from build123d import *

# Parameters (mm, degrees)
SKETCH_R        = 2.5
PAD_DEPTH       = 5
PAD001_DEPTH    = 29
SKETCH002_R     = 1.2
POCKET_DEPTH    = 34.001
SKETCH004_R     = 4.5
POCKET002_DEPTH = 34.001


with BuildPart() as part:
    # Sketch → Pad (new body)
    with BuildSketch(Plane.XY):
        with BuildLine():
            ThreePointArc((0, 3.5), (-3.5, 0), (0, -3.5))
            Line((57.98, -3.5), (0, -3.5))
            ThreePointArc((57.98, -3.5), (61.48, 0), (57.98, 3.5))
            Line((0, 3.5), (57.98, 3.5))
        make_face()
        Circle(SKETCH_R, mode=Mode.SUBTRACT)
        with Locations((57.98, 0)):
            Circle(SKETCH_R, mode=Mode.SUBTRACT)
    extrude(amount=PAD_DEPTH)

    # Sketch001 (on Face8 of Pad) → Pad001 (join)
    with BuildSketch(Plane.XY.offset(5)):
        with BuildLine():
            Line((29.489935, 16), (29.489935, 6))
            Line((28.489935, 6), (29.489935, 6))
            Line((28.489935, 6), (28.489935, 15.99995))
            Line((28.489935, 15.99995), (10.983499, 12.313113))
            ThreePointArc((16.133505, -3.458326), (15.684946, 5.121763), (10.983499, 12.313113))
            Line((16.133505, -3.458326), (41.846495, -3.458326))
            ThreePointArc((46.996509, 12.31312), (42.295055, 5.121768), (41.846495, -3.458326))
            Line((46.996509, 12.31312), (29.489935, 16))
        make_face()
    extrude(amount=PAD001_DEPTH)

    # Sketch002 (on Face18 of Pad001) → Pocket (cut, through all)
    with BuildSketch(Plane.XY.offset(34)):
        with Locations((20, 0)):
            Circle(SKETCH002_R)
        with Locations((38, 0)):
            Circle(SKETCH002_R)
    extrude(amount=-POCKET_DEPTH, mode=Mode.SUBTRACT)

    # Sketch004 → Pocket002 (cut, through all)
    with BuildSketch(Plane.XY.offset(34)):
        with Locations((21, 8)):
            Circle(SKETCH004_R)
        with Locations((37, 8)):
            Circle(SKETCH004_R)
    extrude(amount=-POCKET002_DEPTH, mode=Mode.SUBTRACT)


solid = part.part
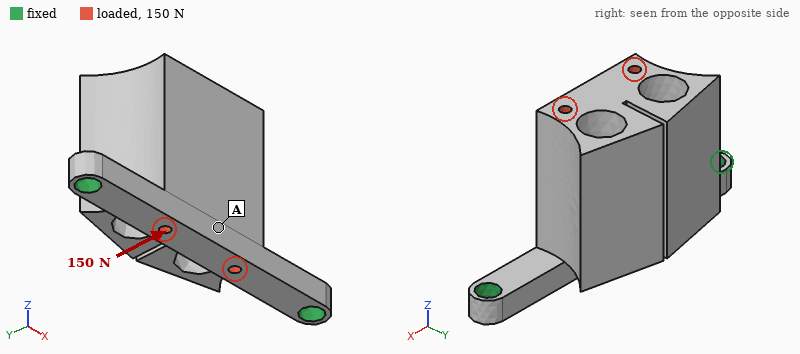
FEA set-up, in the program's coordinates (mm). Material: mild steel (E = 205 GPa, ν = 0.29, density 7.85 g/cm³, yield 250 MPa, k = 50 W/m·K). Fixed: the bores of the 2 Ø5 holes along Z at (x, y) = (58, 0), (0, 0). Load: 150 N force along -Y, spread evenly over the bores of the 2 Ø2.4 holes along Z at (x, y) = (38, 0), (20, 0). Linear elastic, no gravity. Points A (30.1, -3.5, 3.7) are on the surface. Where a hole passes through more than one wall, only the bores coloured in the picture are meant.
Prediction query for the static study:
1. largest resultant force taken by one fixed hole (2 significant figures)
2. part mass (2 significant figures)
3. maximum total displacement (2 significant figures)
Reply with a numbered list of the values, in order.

1. 75 N
2. 97 g
3. 51 µm
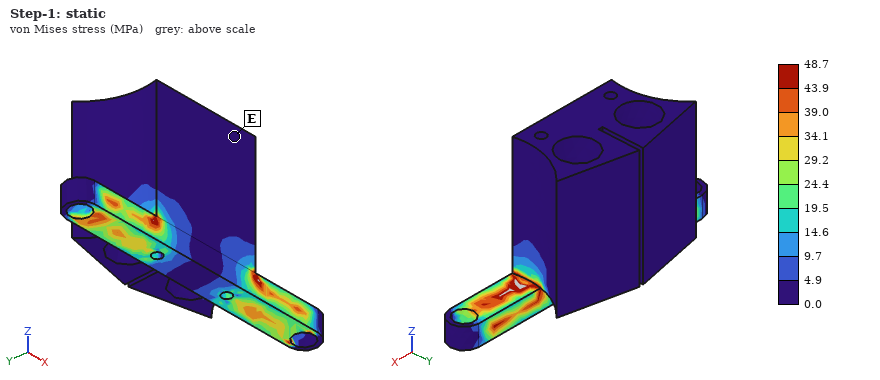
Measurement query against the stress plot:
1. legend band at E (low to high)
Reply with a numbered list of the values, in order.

1. 0.0 to 4.9 MPa
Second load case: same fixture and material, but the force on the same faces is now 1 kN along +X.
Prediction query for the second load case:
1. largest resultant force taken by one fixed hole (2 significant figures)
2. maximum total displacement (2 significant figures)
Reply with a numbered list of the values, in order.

1. 620 N
2. 26 µm
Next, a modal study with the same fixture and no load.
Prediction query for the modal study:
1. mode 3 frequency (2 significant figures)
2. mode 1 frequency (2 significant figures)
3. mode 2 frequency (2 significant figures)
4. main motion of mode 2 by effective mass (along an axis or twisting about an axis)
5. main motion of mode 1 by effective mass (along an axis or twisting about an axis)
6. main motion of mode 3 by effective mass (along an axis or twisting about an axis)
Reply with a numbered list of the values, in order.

1. 4000 Hz
2. 1100 Hz
3. 3700 Hz
4. along X
5. along Y
6. along Z
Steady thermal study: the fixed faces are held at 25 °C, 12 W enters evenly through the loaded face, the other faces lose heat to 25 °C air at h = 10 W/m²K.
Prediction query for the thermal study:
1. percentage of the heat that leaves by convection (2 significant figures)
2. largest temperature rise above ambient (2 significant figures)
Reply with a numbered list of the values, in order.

1. 26 %
2. 55 K
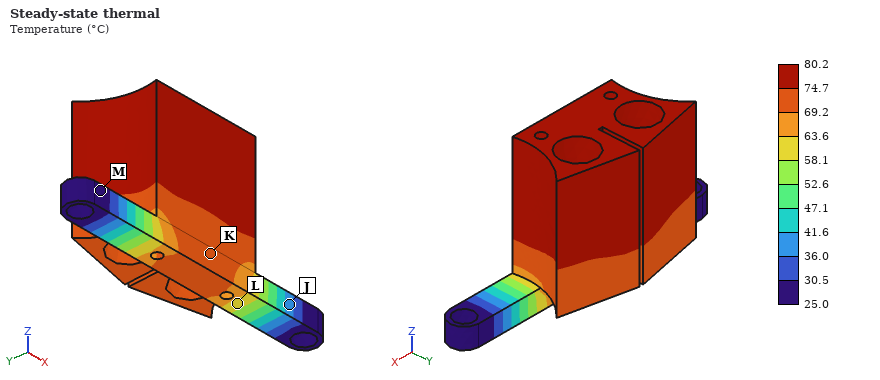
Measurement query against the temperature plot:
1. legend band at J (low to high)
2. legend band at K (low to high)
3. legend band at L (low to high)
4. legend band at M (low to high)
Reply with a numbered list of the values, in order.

1. 36.0 to 41.6 °C
2. 69.2 to 74.7 °C
3. 58.1 to 63.6 °C
4. 25.0 to 30.5 °C
